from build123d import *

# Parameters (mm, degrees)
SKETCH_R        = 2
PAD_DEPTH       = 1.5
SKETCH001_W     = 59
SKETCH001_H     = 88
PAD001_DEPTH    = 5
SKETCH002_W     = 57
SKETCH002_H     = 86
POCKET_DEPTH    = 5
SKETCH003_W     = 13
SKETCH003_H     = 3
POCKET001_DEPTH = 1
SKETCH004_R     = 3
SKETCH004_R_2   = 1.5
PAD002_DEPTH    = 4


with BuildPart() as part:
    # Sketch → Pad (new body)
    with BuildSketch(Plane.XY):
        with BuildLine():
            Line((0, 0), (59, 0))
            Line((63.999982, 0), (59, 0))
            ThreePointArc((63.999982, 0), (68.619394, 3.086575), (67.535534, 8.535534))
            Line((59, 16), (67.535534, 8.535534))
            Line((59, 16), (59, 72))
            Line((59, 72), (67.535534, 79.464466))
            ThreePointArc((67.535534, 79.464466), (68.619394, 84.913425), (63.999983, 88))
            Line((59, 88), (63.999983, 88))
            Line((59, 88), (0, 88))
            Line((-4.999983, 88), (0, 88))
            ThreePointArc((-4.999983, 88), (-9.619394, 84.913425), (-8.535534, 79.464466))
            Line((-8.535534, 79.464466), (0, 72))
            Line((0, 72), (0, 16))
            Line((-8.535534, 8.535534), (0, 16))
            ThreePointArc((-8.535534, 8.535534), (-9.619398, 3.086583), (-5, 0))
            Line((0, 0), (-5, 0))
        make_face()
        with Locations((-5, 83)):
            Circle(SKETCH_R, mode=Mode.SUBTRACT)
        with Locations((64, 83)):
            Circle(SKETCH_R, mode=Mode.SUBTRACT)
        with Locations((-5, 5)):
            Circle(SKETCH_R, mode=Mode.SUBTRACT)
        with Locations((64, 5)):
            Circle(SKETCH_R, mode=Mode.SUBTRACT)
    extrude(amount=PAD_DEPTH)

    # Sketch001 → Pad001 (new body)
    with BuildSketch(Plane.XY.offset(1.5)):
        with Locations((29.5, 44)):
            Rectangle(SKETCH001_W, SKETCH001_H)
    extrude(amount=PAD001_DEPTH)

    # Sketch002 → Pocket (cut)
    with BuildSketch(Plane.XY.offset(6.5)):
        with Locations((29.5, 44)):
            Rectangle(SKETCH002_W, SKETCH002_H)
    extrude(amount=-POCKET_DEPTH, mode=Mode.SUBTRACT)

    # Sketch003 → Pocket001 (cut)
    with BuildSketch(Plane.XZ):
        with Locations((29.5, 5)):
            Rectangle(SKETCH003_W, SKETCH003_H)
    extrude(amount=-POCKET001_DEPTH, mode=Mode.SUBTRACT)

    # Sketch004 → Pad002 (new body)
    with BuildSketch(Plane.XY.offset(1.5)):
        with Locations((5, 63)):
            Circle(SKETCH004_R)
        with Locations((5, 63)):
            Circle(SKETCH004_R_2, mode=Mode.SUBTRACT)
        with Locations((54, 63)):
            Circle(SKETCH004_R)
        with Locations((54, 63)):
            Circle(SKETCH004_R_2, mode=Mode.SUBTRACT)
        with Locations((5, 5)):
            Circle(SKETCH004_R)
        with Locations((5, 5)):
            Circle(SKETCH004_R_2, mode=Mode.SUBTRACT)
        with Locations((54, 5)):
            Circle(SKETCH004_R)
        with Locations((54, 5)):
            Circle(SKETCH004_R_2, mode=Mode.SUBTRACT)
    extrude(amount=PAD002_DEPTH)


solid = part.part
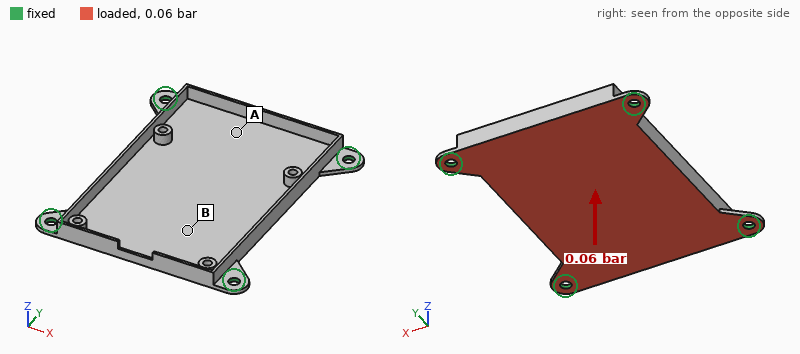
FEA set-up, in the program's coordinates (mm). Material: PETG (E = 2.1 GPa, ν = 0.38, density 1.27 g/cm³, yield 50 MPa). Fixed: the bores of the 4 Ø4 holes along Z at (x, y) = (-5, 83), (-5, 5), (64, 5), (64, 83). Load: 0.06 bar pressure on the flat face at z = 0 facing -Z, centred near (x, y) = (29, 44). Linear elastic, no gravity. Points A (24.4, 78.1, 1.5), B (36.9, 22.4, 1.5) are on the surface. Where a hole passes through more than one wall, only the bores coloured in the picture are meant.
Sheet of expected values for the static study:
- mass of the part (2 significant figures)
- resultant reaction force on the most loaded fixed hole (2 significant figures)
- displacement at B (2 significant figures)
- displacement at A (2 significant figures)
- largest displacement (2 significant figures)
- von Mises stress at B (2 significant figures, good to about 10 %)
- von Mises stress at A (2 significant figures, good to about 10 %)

13 g
11 N
0.83 mm
0.44 mm
1.1 mm
3.1 MPa
1.9 MPa
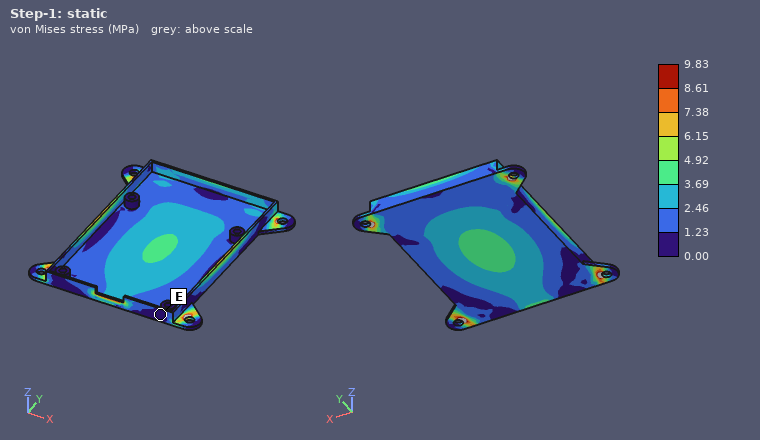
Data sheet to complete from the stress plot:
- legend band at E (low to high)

0.00 to 1.23 MPa
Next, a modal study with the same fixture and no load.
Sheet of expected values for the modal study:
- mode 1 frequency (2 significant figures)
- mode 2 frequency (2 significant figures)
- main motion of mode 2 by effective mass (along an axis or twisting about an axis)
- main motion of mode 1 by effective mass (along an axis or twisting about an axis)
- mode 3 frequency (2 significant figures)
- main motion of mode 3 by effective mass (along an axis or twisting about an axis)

330 Hz
580 Hz
twisting about X
along Z
700 Hz
twisting about Y
